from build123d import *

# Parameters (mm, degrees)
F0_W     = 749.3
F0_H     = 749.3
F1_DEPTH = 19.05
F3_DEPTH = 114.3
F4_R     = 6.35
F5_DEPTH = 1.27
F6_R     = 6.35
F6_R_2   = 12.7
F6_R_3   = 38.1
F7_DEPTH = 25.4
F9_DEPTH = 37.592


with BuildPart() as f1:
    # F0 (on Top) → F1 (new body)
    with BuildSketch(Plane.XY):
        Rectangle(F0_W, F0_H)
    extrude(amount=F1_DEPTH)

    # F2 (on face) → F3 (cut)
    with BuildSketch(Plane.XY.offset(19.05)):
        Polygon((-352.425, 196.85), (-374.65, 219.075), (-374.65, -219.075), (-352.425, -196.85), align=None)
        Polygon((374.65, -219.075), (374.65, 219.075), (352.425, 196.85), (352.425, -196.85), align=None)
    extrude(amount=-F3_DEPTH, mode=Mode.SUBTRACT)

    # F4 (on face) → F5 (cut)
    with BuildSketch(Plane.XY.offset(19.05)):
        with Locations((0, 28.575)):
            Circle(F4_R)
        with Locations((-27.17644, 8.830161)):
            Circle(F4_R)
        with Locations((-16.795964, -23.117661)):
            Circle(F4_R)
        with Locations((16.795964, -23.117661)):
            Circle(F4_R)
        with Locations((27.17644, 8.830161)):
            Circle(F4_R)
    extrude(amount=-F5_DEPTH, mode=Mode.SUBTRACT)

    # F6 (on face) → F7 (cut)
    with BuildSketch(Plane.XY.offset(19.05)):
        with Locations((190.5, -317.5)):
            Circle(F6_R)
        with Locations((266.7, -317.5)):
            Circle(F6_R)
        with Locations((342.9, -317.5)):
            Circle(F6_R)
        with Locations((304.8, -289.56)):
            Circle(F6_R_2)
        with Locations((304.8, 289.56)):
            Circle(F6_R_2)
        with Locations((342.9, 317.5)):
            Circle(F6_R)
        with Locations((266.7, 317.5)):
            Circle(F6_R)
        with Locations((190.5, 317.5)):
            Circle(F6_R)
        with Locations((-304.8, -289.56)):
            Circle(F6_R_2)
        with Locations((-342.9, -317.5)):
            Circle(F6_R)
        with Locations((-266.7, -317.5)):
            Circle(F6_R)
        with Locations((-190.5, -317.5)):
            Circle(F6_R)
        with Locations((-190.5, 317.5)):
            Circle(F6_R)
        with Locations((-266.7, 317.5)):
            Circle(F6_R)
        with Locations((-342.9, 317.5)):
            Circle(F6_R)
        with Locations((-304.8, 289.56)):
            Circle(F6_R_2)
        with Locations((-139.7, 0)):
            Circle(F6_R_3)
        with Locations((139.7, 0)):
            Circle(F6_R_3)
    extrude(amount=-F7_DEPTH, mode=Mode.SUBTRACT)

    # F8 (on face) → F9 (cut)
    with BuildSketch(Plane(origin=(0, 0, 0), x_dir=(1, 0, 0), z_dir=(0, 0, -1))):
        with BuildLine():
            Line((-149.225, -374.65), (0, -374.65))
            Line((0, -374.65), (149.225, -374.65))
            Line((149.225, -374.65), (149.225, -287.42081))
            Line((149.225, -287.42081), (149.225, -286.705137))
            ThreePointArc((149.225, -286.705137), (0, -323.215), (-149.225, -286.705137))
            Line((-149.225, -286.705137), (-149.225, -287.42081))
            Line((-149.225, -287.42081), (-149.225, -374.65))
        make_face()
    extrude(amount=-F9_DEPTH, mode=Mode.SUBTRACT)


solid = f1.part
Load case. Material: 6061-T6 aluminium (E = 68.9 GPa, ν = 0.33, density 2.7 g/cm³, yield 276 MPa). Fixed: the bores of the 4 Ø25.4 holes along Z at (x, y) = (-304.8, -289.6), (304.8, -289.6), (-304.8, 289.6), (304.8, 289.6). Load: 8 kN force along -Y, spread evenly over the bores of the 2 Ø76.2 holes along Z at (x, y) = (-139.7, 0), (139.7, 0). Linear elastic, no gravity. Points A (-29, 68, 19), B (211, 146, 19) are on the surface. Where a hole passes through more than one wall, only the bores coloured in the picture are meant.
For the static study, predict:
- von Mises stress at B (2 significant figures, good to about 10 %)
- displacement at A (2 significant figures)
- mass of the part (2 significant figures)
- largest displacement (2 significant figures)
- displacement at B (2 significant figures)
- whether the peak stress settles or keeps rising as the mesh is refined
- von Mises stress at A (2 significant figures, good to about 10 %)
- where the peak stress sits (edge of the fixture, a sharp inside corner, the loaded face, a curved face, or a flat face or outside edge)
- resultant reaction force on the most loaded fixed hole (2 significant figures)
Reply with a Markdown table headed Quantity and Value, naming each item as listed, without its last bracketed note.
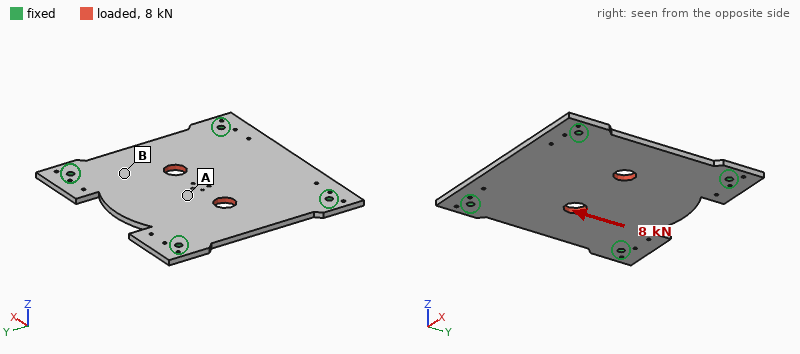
| Quantity | Value |
|---|---|
| von Mises stress at B | 0.65 MPa |
| displacement at A | 3.7 µm |
| mass of the part | 26 kg |
| largest displacement | 4.5 µm |
| displacement at B | 2.4 µm |
| whether the peak stress settles or keeps rising as the mesh is refined | keeps rising |
| von Mises stress at A | 0.22 MPa |
| where the peak stress sits | edge of the fixture |
| resultant reaction force on the most loaded fixed hole | 2.2 kN |
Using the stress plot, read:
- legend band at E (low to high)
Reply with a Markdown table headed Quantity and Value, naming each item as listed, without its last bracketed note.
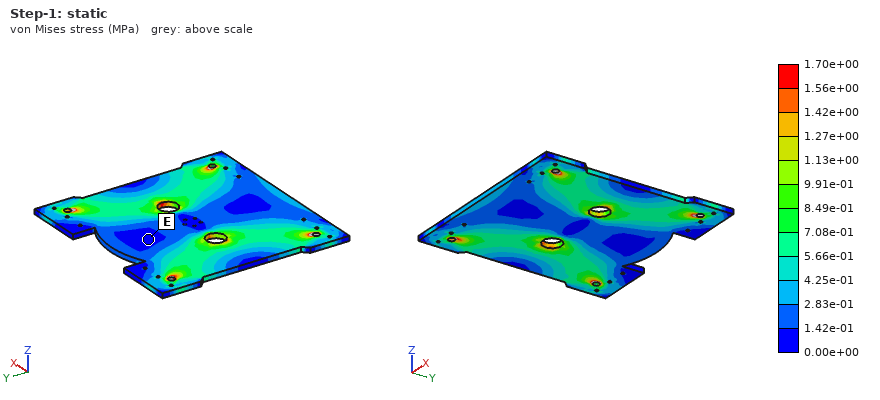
| Quantity | Value |
|---|---|
| legend band at E | 0.00e+00 to 1.42e-01 MPa |
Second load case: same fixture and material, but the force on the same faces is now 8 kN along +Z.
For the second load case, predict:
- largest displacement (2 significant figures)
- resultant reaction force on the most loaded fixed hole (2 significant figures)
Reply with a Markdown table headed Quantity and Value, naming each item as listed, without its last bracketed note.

| Quantity | Value |
|---|---|
| largest displacement | 0.78 mm |
| resultant reaction force on the most loaded fixed hole | 2.0 kN |
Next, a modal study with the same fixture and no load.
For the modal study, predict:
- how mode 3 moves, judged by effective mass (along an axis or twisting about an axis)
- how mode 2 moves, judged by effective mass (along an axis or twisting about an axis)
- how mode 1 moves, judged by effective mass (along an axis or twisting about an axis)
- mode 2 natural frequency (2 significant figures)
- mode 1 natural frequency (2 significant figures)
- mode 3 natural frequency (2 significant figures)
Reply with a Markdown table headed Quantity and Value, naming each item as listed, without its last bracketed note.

| Quantity | Value |
|---|---|
| how mode 3 moves, judged by effective mass | twisting about Y |
| how mode 2 moves, judged by effective mass | twisting about X |
| how mode 1 moves, judged by effective mass | along Z |
| mode 2 natural frequency | 290 Hz |
| mode 1 natural frequency | 180 Hz |
| mode 3 natural frequency | 330 Hz |
